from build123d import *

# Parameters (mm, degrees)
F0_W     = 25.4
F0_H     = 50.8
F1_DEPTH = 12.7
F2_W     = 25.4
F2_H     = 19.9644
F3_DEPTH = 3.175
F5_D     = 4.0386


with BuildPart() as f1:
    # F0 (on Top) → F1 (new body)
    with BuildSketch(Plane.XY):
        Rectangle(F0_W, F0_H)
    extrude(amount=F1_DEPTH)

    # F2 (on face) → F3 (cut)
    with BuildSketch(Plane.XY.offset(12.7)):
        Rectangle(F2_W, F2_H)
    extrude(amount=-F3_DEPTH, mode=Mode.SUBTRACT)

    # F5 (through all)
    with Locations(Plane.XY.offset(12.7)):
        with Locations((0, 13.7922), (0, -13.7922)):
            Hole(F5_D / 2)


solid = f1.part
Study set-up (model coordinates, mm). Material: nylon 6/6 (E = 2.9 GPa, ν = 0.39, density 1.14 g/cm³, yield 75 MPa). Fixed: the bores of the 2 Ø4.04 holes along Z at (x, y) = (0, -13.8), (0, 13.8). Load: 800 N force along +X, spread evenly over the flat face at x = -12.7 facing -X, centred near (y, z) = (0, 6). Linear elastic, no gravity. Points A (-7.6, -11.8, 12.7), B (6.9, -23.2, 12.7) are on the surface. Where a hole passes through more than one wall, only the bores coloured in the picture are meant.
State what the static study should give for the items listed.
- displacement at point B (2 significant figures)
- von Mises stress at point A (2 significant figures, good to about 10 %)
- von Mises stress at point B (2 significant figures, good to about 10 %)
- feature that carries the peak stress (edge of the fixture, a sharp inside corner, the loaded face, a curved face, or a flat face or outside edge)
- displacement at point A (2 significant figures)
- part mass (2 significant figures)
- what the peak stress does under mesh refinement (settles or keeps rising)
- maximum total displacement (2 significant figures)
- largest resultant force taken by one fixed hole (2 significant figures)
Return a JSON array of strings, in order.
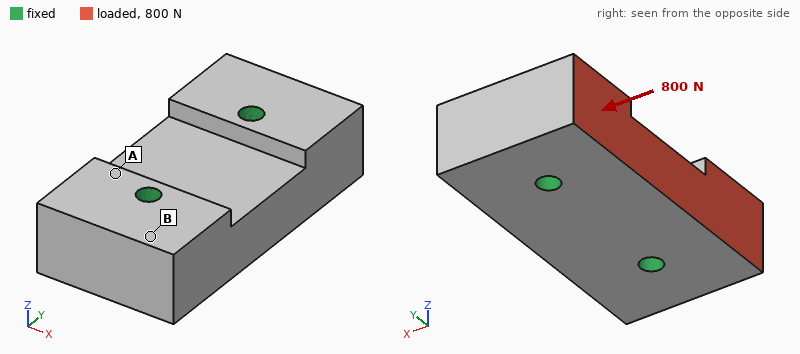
["6.1 µm", "1.5 MPa", "0.48 MPa", "edge of the fixture", "4.0 µm", "16 g", "keeps rising", "16 µm", "400 N"]
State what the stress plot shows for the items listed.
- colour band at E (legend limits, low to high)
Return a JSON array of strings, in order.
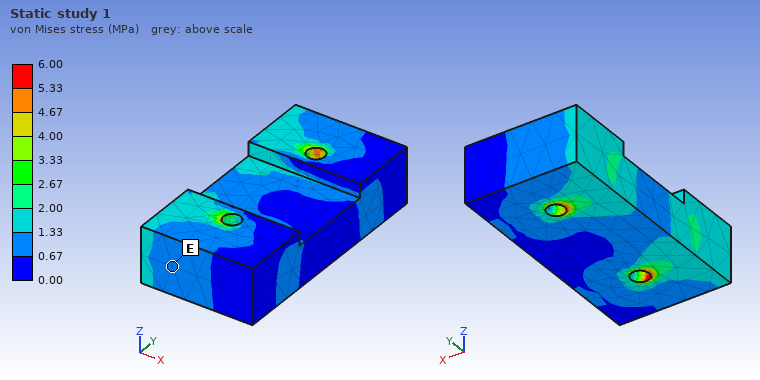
["0.67 to 1.33 MPa"]
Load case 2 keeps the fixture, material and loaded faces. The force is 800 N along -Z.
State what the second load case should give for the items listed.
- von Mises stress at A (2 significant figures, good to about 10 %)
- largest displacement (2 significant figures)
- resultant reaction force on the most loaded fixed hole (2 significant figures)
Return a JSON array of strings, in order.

["4.3 MPa", "83 µm", "400 N"]
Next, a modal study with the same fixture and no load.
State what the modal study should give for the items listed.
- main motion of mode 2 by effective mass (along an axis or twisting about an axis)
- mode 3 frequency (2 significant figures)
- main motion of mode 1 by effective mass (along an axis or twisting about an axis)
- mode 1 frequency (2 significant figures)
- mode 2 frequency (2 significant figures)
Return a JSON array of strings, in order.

["twisting about Z", "10 kHz", "twisting about Y", "9000 Hz", "9700 Hz"]
